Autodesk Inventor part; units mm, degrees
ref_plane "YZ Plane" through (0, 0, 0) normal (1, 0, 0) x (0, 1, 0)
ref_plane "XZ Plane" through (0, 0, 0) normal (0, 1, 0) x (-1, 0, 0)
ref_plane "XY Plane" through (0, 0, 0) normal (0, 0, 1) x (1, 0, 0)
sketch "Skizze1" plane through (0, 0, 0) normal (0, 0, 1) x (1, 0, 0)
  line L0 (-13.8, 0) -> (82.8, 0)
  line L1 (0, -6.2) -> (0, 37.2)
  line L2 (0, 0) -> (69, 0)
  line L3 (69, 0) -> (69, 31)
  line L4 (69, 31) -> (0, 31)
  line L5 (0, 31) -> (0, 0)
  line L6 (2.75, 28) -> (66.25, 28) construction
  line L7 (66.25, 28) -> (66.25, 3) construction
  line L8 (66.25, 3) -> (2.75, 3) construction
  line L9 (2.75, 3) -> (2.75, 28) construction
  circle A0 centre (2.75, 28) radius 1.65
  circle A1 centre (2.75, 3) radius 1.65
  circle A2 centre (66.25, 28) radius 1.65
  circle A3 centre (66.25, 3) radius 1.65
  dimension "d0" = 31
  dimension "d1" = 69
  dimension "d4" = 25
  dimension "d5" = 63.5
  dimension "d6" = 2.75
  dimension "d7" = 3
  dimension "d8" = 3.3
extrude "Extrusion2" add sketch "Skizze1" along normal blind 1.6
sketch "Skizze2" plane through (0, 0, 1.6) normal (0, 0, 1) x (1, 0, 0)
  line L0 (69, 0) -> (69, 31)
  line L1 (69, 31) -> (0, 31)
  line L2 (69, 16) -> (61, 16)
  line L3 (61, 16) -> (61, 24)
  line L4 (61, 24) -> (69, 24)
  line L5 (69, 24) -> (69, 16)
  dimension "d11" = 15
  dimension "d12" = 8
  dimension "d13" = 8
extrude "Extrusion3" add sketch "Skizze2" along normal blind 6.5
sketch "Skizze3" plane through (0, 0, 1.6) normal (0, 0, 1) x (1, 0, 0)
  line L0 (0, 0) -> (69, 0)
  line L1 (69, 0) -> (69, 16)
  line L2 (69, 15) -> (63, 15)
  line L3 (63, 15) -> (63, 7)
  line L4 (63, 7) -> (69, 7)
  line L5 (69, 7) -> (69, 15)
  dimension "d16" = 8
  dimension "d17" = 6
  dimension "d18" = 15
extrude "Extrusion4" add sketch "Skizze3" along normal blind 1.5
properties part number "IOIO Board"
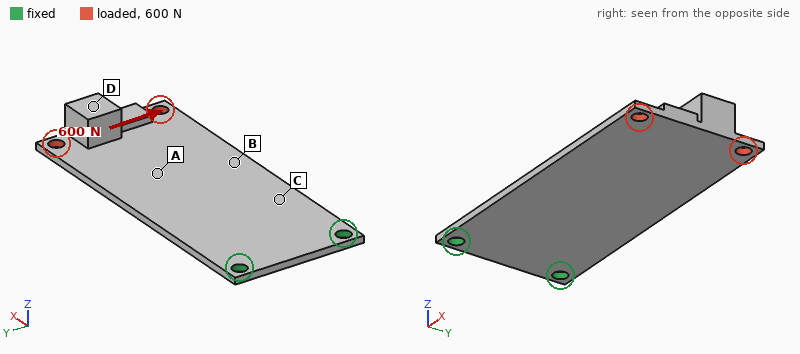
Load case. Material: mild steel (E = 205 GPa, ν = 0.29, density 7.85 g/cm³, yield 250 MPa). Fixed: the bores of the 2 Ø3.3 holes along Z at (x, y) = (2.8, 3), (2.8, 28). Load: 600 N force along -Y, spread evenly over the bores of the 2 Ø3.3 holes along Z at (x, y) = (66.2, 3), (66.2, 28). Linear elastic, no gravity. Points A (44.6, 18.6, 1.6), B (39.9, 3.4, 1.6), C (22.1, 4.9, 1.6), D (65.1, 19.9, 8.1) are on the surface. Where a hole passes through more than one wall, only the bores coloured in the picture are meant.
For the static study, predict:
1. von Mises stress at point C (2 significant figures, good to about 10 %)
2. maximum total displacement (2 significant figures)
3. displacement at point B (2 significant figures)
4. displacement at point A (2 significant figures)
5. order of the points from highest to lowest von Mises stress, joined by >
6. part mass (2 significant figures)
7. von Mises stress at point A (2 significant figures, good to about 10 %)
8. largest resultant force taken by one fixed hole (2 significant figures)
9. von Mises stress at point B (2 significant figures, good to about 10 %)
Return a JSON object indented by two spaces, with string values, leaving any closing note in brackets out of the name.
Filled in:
{
  "von Mises stress at point C": "73 MPa",
  "maximum total displacement": "83 µm",
  "displacement at point B": "36 µm",
  "displacement at point A": "39 µm",
  "order of the points from highest to lowest von Mises stress, joined by >": "C > B > A > D",
  "part mass": "30 g",
  "von Mises stress at point A": "32 MPa",
  "largest resultant force taken by one fixed hole": "1.5 kN",
  "von Mises stress at point B": "50 MPa"
}
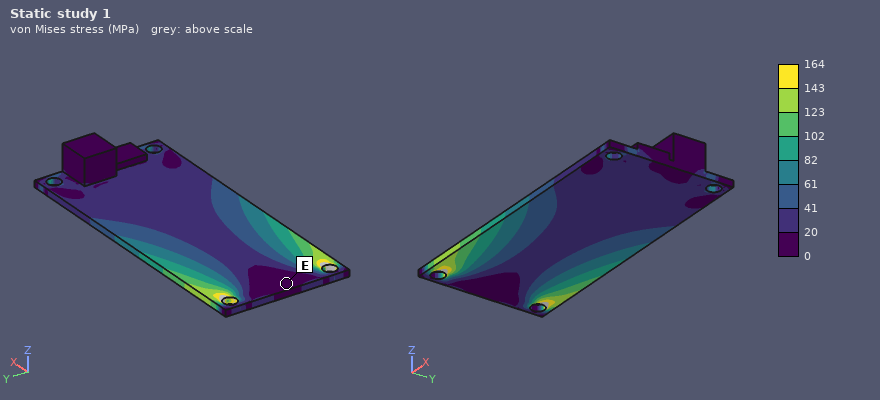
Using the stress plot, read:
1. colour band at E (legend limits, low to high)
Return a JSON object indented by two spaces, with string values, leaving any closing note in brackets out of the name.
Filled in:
{
  "colour band at E": "0 to 20 MPa"
}
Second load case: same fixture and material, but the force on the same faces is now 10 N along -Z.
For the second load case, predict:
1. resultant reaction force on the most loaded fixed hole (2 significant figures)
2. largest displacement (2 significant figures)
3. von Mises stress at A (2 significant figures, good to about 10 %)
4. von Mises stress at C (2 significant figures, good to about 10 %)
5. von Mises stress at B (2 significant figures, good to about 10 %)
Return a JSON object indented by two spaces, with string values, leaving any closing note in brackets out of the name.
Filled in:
{
  "resultant reaction force on the most loaded fixed hole": "5.0 N",
  "largest displacement": "0.44 mm",
  "von Mises stress at A": "16 MPa",
  "von Mises stress at C": "33 MPa",
  "von Mises stress at B": "20 MPa"
}
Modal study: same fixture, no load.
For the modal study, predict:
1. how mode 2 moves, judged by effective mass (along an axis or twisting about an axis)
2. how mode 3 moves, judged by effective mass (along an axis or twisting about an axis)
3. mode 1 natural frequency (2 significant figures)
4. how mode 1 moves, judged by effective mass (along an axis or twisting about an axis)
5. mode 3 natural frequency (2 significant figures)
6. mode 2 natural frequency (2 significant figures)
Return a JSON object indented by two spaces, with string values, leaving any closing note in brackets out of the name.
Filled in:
{
  "how mode 2 moves, judged by effective mass": "twisting about X",
  "how mode 3 moves, judged by effective mass": "along Z",
  "mode 1 natural frequency": "240 Hz",
  "how mode 1 moves, judged by effective mass": "along Z",
  "mode 3 natural frequency": "1700 Hz",
  "mode 2 natural frequency": "1300 Hz"
}
